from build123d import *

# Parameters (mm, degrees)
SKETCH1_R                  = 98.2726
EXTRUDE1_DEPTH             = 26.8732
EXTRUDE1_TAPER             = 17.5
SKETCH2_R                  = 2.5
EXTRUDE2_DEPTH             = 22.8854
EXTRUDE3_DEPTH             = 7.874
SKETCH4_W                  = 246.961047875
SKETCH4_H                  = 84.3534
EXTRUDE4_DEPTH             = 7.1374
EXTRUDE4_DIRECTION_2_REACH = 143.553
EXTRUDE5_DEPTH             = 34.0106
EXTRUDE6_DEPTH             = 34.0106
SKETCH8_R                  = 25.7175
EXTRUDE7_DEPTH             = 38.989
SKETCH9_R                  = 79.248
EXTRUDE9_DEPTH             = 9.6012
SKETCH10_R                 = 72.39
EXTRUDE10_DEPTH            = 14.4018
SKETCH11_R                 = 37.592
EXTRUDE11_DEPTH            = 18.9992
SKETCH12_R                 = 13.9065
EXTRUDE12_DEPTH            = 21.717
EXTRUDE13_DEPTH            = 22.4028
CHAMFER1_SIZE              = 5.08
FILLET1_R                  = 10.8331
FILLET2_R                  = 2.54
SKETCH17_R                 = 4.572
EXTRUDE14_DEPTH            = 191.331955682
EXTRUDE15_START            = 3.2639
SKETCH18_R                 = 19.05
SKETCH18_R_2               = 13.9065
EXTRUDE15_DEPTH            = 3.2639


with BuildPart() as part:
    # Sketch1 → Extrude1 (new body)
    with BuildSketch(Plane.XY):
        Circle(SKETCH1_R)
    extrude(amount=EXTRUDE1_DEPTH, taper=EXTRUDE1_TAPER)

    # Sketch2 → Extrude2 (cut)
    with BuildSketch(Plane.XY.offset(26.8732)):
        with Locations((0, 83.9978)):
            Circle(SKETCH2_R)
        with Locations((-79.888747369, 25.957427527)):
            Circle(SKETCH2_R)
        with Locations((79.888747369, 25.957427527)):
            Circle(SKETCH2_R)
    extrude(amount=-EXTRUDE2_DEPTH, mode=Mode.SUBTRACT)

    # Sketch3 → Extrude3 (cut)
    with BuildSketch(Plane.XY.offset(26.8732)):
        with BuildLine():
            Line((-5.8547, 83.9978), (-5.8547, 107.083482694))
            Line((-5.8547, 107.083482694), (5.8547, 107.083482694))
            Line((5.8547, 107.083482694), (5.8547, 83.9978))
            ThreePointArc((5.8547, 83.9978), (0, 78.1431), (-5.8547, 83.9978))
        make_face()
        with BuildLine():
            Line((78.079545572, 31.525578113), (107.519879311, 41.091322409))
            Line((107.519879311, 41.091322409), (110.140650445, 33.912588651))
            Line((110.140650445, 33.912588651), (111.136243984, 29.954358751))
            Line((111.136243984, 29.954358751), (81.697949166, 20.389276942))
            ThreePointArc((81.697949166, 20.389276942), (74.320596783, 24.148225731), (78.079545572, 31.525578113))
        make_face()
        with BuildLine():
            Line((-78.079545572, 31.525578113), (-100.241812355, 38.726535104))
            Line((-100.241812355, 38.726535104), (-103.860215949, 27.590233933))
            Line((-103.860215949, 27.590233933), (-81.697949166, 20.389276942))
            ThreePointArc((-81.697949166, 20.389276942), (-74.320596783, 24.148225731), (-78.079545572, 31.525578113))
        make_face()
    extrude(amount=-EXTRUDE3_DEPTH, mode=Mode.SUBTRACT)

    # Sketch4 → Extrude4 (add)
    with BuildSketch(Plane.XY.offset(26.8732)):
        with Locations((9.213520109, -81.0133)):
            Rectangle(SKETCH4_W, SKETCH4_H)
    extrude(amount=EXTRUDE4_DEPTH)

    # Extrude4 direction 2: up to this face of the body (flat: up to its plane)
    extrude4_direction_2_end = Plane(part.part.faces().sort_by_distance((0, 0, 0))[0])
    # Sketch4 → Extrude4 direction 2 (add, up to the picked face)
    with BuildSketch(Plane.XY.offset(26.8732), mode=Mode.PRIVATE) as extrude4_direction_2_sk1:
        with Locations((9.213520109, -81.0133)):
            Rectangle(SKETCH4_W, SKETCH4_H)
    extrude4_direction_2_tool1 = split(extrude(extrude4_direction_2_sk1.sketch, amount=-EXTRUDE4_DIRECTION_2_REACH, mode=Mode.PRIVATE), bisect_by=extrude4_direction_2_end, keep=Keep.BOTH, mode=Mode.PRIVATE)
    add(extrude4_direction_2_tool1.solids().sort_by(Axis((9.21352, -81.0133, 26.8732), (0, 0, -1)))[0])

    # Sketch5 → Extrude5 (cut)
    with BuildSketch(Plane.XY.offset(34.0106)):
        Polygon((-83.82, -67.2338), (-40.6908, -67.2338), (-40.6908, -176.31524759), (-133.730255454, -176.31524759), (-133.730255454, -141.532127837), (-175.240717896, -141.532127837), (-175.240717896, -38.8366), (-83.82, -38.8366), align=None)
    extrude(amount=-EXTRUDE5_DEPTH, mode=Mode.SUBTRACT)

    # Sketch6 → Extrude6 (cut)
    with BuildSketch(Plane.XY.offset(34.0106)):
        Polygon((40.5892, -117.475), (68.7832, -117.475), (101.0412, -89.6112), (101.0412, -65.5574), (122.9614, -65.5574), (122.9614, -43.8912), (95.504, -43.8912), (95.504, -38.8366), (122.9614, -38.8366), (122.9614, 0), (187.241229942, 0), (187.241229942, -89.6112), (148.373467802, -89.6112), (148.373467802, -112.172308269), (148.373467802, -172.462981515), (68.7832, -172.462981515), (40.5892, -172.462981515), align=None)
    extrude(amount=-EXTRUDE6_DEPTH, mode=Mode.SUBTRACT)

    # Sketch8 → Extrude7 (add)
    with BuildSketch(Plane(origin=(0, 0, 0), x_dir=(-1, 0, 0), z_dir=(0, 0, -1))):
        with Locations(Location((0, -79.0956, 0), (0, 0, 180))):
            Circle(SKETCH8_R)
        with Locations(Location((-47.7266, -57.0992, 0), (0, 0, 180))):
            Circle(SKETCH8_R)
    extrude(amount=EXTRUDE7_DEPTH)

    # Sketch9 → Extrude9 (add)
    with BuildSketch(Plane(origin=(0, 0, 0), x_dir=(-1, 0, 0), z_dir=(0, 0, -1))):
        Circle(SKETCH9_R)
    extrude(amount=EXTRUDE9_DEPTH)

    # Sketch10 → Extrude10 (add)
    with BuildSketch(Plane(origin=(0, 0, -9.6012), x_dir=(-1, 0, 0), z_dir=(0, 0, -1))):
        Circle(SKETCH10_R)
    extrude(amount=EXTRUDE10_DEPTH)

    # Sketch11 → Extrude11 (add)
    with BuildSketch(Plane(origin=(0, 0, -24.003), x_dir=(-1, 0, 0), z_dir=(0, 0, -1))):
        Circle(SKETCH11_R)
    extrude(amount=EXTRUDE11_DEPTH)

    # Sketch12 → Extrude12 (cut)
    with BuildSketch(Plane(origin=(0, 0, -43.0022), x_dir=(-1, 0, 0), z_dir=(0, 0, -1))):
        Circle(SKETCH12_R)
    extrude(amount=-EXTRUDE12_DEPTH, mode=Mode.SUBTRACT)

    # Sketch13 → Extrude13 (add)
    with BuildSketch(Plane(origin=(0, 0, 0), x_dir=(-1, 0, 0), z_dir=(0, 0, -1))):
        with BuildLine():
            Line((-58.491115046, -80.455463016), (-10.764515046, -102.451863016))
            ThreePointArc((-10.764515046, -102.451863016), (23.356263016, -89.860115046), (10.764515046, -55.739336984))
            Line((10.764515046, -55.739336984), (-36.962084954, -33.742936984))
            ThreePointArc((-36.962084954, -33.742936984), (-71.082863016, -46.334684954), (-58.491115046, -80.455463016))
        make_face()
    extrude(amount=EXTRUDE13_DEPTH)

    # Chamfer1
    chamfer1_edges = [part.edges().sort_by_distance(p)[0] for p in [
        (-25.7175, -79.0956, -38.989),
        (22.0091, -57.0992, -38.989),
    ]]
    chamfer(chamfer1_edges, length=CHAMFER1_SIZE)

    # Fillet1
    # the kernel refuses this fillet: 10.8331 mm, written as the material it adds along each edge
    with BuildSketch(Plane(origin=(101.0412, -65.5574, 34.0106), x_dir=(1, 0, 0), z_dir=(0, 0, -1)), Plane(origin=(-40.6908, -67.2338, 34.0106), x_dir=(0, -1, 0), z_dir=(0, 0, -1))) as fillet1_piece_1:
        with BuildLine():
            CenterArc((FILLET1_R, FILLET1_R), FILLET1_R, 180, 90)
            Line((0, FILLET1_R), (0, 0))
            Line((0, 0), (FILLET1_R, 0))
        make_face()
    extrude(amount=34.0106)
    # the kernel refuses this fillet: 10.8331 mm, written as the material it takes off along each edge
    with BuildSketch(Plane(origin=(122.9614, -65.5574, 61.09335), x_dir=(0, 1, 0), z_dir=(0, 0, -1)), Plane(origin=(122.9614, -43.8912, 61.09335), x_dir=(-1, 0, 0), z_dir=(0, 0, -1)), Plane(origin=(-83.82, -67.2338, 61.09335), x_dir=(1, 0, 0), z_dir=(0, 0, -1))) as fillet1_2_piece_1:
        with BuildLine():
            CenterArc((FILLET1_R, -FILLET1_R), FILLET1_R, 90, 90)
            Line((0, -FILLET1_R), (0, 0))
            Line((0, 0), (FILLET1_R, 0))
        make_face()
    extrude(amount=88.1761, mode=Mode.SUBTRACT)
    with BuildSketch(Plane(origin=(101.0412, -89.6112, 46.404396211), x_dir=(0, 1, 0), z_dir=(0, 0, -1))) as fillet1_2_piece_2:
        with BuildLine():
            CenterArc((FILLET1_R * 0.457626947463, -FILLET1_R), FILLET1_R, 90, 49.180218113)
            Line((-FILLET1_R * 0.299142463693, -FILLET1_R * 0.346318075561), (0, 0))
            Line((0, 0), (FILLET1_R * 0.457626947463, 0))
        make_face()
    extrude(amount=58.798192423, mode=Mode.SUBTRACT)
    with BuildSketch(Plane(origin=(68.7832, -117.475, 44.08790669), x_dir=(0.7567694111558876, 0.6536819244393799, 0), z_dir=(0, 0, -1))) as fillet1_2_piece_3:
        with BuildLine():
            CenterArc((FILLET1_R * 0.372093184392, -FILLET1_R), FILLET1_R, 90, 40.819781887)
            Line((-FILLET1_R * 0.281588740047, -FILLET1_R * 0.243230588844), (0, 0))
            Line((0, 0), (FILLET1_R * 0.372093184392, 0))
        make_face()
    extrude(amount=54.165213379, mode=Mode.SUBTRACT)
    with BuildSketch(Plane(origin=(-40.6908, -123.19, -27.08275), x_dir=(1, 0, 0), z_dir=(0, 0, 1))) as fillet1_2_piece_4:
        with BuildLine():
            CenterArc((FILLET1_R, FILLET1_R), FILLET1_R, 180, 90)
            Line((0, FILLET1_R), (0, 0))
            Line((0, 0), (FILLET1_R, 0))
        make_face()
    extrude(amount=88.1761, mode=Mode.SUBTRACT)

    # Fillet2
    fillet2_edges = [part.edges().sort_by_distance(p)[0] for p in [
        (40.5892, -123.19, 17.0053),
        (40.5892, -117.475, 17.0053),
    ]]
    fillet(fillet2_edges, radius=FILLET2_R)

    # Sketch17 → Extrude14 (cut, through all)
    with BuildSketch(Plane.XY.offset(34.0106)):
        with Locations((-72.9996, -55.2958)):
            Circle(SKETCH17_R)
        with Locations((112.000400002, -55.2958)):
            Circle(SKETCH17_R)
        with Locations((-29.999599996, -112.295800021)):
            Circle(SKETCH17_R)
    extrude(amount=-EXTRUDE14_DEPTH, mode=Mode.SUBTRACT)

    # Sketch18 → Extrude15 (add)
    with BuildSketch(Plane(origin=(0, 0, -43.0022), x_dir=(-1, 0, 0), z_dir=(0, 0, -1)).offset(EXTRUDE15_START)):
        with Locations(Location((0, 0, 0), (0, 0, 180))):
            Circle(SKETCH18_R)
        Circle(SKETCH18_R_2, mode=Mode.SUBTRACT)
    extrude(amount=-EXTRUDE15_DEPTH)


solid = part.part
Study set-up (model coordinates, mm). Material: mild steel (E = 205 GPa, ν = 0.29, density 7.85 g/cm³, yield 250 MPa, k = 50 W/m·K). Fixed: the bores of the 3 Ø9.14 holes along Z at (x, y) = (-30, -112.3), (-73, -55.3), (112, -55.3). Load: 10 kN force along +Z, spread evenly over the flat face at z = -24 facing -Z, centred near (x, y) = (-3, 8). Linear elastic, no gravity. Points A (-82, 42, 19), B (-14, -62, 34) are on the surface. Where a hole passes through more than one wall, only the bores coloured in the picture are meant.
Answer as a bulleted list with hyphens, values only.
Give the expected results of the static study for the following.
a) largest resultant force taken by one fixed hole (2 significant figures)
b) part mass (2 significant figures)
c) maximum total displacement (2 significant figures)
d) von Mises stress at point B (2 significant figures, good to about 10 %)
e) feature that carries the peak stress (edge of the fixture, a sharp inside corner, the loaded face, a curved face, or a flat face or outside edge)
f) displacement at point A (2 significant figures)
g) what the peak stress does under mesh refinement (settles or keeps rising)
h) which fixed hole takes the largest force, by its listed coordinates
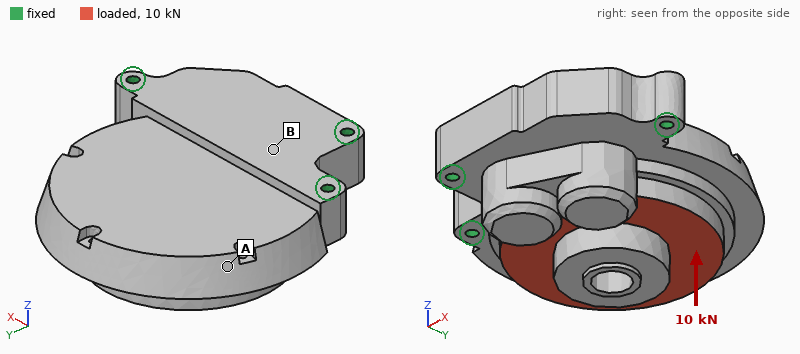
- 10 kN
- 13 kg
- 44 µm
- 9.3 MPa
- edge of the fixture
- 24 µm
- keeps rising
- (-73, -55.3)
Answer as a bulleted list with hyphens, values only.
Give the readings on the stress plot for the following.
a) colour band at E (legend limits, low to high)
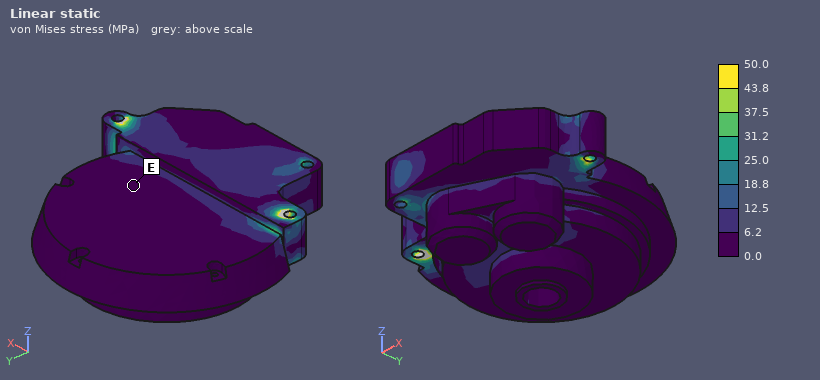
- 0.0 to 6.2 MPa
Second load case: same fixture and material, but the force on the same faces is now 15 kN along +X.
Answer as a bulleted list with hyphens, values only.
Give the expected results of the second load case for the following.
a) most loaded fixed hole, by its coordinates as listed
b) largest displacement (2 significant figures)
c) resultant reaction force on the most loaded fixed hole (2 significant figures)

- (-73, -55.3)
- 9.3 µm
- 11 kN
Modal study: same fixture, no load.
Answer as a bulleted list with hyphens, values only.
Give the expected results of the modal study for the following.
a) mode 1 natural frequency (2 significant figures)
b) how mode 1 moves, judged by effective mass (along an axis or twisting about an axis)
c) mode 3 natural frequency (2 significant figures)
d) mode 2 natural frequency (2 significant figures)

- 1000 Hz
- along Z
- 3300 Hz
- 2700 Hz
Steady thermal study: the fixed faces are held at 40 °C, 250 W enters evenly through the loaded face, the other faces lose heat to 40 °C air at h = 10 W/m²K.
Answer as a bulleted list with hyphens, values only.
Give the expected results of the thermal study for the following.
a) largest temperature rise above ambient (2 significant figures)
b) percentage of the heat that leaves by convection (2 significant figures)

- 72 K
- 18 %
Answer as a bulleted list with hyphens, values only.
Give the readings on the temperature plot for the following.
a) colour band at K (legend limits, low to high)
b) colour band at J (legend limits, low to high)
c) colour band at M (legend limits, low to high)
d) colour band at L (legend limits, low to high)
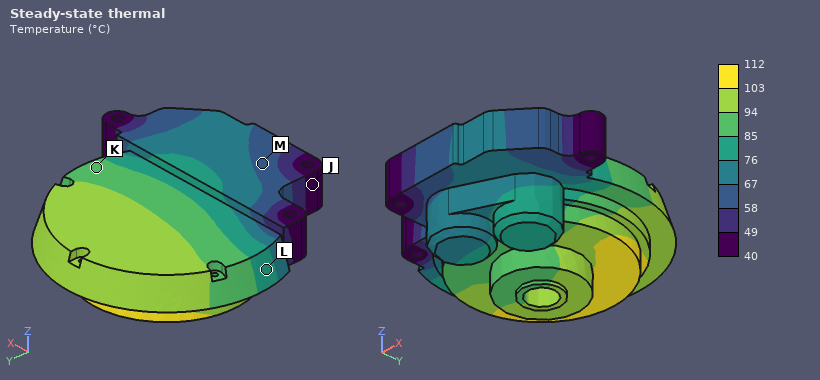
- 85 to 94 °C
- 40 to 49 °C
- 58 to 67 °C
- 76 to 85 °C
